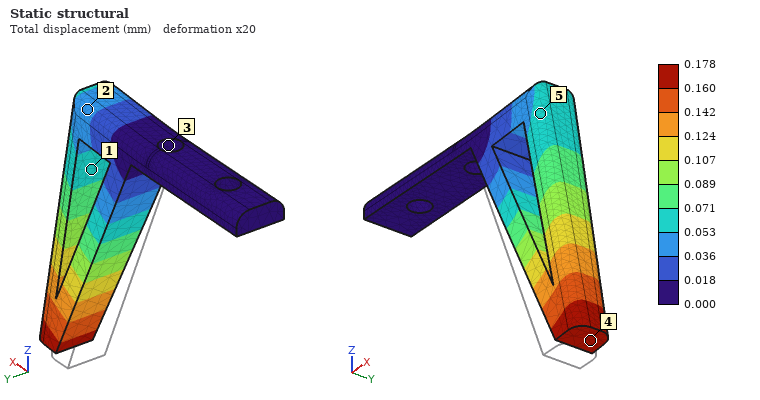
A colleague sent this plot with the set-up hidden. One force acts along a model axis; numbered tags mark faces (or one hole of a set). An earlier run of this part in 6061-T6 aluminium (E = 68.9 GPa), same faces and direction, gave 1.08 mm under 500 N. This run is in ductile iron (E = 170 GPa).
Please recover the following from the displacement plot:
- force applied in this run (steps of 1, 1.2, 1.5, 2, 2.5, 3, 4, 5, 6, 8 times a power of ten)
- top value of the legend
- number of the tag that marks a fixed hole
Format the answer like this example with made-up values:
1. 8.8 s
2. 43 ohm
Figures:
1. 200 N
2. 0.178 mm
3. 3
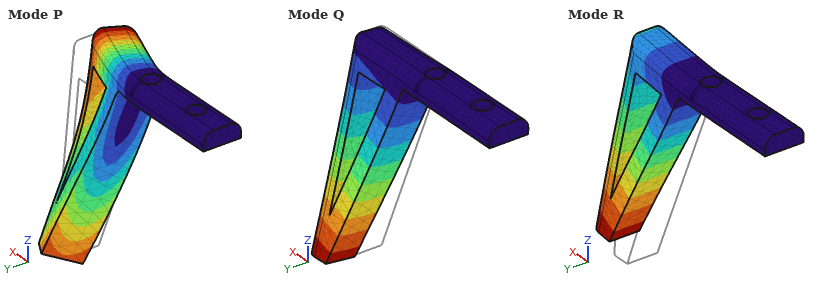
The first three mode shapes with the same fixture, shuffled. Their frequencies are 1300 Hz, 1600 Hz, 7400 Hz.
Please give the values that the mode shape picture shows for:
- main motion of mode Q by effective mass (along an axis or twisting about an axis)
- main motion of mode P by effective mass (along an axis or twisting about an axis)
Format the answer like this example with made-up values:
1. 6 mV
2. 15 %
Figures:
1. along Y
2. along Y
